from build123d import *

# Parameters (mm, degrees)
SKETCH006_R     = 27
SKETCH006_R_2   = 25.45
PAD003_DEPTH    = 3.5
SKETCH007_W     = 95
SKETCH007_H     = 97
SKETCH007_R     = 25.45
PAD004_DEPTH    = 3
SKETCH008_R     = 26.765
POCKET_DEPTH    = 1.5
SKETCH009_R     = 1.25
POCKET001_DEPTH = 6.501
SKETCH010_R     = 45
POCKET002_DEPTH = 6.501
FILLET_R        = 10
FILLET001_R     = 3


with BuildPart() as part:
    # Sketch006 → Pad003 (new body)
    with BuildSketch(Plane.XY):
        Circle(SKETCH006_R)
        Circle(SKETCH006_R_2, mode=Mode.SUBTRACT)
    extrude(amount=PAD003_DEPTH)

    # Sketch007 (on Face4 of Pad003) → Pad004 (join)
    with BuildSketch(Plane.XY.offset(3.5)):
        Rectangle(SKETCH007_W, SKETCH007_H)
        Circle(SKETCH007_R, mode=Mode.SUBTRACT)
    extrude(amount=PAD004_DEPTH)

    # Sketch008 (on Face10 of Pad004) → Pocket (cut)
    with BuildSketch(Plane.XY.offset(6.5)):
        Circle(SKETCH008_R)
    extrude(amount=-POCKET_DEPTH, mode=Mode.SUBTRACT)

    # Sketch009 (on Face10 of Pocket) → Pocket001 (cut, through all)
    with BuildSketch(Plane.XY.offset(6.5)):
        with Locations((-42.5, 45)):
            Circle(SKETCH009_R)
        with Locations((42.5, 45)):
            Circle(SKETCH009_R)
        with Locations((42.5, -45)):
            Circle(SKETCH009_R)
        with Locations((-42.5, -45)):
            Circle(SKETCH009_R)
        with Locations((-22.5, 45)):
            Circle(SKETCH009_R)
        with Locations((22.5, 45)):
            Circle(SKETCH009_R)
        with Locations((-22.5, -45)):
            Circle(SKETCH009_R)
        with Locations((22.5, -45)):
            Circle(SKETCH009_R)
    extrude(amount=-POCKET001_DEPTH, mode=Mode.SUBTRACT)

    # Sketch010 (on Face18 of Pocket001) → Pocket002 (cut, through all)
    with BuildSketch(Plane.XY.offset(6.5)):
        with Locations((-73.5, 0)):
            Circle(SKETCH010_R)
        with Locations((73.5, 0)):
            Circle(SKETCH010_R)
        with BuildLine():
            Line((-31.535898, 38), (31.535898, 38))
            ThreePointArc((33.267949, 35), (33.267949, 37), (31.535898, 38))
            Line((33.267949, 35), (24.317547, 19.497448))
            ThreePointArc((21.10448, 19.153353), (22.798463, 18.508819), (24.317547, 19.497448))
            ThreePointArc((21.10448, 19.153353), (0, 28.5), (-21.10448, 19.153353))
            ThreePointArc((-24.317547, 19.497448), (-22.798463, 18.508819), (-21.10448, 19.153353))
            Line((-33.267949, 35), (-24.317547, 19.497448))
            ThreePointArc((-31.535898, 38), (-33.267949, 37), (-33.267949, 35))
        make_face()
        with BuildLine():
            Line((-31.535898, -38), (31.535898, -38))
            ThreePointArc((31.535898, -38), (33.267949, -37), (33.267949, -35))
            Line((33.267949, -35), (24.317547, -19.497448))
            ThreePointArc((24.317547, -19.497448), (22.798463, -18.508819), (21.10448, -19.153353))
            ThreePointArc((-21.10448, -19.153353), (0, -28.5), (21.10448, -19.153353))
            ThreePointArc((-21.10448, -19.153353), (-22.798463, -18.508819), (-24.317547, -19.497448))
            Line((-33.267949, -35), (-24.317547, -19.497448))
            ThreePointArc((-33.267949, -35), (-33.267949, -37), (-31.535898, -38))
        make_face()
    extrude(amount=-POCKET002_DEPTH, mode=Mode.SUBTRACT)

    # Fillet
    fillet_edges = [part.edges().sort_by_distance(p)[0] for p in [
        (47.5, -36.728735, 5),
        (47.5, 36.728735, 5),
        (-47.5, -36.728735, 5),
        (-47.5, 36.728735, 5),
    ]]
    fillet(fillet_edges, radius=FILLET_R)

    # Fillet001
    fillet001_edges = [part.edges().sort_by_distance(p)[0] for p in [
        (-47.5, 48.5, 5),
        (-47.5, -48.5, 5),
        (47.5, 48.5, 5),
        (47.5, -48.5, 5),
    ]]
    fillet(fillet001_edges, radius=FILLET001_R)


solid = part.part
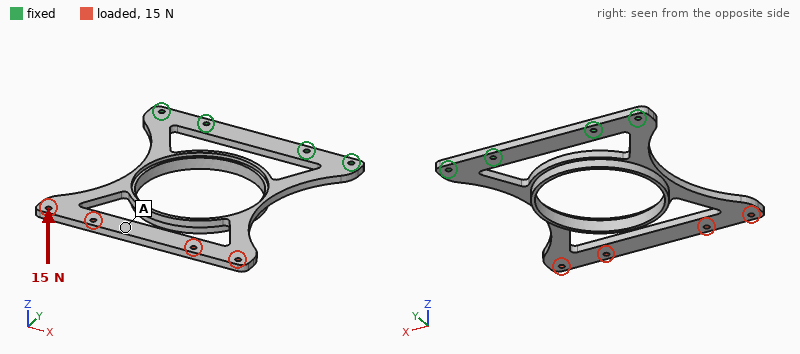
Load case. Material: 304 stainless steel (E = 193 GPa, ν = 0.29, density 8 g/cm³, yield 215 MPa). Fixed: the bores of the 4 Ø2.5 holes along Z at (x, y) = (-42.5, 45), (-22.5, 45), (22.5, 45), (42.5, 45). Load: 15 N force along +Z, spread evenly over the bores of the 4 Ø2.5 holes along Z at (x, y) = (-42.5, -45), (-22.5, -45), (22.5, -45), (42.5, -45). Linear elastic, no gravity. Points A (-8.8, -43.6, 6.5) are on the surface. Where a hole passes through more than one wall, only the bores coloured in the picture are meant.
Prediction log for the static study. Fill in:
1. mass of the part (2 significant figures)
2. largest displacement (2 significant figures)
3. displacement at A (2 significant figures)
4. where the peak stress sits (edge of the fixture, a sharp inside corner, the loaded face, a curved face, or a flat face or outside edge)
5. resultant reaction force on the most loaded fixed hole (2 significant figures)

88 g
0.48 mm
0.44 mm
a curved face
8.4 N
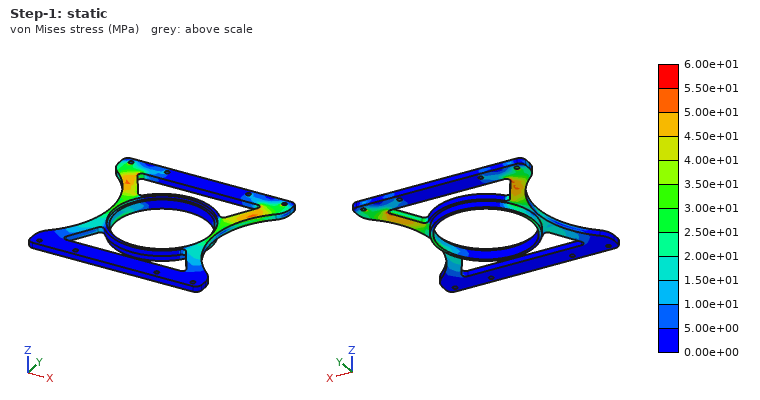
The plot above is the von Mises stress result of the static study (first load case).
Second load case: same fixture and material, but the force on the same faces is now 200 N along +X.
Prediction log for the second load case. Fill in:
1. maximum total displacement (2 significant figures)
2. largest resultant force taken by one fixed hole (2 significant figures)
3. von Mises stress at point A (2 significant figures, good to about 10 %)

0.25 mm
250 N
13 MPa
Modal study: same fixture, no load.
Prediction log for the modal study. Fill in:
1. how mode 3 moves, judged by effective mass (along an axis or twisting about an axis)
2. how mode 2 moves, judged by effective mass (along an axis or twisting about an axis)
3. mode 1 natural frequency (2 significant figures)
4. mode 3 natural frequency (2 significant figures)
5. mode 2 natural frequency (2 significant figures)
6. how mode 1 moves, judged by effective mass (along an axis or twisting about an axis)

along X
twisting about Y
160 Hz
810 Hz
390 Hz
along Z
